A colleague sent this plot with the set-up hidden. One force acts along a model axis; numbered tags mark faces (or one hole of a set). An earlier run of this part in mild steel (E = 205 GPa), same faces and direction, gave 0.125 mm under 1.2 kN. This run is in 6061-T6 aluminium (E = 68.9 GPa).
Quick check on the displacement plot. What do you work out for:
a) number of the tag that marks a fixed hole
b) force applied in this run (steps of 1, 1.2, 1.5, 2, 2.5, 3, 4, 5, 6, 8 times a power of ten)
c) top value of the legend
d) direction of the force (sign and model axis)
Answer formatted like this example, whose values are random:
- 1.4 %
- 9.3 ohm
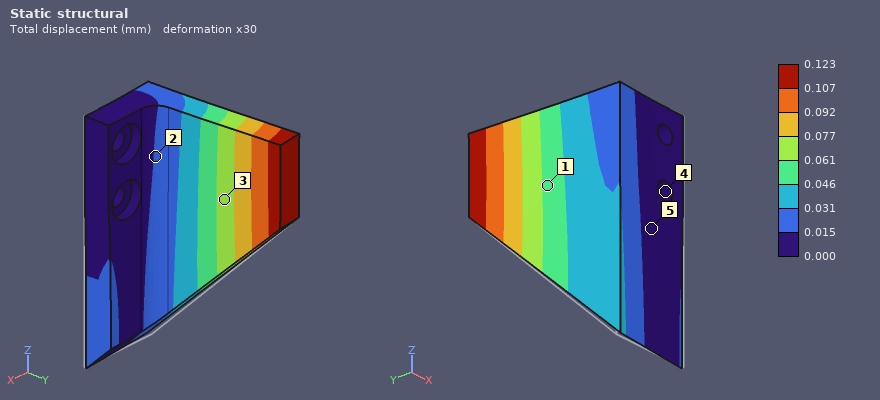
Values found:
- 4
- 400 N
- 0.123 mm
- -X
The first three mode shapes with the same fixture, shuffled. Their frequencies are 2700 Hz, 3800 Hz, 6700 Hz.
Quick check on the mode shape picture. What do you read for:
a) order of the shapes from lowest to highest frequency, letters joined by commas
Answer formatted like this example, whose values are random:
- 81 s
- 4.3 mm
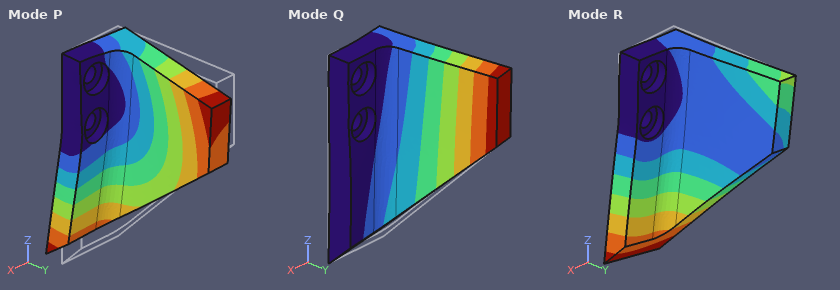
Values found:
- Q, P, R
